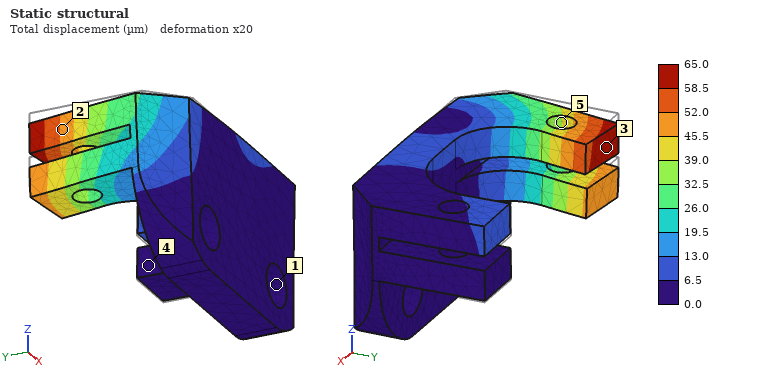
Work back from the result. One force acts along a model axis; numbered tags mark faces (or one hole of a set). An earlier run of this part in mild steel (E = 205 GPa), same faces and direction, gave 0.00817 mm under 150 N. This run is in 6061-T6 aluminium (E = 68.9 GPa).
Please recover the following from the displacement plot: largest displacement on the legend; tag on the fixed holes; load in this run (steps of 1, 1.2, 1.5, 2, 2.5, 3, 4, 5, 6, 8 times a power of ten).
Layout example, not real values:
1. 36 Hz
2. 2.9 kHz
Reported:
1. 65.0 µm
2. 1
3. 400 N
